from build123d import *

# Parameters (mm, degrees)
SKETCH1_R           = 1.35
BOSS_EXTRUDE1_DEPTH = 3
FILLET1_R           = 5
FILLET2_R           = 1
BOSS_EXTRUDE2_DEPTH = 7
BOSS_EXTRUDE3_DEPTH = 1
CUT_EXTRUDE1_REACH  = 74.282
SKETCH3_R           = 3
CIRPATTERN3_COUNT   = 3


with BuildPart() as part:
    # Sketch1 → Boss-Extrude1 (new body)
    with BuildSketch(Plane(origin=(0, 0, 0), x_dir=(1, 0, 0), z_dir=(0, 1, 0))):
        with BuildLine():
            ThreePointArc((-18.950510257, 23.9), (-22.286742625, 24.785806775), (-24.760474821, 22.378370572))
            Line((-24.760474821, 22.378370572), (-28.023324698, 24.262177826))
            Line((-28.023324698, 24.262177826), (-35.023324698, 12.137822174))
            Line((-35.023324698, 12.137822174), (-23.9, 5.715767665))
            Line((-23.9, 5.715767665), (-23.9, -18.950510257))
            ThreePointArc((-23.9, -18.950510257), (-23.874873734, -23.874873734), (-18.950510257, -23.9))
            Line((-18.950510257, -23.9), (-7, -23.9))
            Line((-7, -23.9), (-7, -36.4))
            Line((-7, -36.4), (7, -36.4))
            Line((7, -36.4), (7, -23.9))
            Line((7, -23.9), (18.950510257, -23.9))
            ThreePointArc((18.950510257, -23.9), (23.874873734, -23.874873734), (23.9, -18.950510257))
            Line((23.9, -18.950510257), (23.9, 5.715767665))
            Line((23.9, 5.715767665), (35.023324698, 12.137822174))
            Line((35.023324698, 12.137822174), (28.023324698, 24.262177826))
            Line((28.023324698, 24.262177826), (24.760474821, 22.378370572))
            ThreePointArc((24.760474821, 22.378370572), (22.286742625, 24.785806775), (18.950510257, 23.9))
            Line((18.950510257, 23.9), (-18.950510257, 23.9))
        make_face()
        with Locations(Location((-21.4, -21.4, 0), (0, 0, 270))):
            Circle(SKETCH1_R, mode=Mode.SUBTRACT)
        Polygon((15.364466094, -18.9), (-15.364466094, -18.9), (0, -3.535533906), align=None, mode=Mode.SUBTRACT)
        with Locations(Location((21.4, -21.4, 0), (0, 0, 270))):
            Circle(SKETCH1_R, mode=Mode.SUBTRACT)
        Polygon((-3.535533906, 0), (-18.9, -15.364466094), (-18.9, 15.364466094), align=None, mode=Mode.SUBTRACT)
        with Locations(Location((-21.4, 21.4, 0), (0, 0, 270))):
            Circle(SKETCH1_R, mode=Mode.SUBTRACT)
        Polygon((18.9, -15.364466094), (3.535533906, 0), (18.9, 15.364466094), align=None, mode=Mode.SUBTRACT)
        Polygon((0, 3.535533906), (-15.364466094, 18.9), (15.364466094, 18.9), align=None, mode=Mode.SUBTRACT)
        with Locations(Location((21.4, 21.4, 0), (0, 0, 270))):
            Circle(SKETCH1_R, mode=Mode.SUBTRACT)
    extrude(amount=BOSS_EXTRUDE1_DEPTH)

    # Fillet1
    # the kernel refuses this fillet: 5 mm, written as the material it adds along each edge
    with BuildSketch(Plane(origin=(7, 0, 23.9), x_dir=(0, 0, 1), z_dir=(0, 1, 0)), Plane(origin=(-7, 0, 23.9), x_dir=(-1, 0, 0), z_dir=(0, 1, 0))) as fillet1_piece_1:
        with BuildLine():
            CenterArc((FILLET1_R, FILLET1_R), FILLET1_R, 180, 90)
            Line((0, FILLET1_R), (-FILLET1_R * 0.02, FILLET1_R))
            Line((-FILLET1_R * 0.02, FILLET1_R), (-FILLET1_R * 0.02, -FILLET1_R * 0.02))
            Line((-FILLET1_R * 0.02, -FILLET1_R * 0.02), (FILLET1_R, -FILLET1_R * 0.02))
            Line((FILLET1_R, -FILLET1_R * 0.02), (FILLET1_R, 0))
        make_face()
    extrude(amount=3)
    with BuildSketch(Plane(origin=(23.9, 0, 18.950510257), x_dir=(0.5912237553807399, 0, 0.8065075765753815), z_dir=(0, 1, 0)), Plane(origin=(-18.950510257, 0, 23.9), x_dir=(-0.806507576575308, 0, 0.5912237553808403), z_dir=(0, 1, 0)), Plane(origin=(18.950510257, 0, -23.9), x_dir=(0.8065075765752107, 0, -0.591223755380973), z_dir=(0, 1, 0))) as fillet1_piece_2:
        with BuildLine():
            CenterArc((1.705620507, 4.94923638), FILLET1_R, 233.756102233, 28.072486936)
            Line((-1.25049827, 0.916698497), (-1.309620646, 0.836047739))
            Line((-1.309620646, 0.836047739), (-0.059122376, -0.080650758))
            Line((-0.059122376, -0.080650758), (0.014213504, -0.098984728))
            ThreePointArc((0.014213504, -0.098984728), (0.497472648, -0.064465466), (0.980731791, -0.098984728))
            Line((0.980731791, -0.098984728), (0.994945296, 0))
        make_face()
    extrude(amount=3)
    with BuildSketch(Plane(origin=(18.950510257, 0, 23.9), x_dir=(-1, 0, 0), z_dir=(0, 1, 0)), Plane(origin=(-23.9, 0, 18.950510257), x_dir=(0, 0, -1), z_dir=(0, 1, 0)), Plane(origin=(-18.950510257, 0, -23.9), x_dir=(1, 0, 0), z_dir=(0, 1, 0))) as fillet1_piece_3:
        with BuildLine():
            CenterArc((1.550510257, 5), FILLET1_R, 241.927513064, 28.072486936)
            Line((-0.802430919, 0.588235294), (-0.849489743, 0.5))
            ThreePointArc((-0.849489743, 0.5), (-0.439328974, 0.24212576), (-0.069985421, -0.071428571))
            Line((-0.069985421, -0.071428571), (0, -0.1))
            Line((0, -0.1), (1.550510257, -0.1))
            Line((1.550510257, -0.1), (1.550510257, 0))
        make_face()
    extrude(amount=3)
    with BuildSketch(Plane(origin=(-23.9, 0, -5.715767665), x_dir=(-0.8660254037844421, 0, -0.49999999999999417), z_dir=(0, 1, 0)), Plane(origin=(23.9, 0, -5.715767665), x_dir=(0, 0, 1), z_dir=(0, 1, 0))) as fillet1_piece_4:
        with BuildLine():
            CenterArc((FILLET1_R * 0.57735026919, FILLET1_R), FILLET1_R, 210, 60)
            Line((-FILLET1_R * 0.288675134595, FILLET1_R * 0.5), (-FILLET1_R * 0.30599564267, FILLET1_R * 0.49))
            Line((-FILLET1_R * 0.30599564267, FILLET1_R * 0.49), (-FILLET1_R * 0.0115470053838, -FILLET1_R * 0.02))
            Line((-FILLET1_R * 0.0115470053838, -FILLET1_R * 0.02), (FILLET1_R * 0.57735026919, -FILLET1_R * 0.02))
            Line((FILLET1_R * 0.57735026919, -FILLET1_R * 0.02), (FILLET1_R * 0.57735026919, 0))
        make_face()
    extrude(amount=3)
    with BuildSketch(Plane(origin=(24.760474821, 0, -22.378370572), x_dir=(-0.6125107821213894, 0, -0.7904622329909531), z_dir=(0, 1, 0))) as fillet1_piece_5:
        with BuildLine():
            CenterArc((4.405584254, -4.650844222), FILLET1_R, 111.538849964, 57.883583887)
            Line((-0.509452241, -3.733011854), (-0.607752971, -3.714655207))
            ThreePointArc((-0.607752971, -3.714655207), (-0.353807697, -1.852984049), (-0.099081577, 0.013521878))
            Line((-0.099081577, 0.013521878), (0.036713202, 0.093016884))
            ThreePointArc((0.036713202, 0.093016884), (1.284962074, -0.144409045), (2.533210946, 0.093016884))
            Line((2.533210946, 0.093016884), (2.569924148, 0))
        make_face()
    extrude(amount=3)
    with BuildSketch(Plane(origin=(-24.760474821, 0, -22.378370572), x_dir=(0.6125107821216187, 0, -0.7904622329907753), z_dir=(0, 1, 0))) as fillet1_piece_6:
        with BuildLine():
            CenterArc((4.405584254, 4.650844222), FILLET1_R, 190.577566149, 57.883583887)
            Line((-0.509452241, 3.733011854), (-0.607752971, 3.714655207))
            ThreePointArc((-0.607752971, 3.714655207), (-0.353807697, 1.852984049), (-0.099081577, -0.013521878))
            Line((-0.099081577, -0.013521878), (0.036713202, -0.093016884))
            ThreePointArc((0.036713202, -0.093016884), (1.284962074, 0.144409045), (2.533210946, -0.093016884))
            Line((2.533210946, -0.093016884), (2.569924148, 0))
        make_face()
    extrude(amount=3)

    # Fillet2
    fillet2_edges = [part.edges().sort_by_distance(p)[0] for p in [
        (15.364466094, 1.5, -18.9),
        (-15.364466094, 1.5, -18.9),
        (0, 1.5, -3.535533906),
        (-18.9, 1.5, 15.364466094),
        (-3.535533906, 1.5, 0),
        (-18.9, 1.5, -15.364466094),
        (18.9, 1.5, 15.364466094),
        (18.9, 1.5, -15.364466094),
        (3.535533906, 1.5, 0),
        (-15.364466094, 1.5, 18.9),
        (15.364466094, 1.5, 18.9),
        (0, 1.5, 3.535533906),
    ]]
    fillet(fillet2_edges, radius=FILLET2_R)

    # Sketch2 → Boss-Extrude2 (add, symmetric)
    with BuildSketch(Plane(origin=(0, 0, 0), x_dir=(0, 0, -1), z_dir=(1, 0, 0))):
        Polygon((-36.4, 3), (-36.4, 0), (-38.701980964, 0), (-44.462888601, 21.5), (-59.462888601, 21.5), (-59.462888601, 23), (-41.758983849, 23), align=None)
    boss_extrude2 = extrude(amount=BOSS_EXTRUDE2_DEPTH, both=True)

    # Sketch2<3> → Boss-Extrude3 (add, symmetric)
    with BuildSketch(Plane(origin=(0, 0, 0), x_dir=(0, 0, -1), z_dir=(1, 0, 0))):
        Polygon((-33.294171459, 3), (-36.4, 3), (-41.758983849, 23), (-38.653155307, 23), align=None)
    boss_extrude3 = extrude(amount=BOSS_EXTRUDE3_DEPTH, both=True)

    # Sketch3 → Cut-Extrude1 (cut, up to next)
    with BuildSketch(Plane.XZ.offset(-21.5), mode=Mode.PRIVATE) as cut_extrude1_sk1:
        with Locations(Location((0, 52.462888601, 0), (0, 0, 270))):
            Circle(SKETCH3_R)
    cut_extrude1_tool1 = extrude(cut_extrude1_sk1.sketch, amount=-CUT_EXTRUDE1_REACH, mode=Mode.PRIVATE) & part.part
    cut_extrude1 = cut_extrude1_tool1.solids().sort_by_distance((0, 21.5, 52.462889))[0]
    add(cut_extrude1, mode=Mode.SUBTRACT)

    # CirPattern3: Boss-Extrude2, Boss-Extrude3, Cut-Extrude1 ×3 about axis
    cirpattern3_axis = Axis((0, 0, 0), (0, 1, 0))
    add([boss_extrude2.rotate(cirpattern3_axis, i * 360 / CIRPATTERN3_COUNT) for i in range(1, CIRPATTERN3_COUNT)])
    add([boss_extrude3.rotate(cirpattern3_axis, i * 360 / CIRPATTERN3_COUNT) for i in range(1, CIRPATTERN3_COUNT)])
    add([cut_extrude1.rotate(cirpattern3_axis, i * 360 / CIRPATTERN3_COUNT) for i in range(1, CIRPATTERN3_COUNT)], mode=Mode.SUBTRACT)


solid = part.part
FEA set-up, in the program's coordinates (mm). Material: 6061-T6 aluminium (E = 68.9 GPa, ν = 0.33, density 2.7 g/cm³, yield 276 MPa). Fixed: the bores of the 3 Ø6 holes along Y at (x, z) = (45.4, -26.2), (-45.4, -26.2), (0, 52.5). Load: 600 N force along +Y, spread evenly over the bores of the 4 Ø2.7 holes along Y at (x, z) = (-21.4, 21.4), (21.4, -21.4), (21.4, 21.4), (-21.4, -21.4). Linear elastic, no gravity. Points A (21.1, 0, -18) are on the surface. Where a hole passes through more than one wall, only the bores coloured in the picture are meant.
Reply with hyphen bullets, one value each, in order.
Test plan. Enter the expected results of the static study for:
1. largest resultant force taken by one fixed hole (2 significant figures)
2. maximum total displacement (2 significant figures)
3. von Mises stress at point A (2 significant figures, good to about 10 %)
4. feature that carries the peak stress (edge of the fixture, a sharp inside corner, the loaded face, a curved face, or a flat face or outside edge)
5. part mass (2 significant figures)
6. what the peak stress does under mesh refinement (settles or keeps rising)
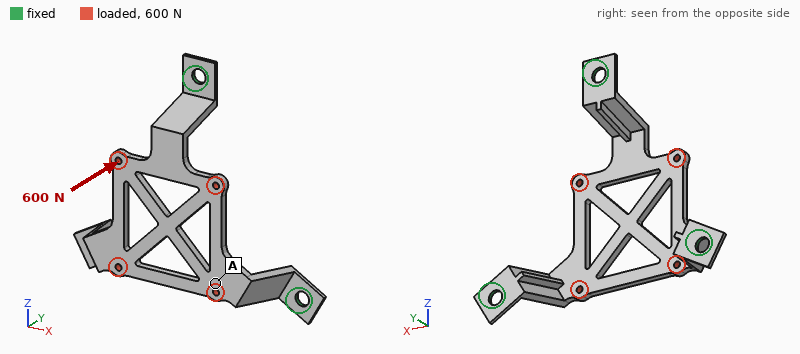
- 280 N
- 0.32 mm
- 27 MPa
- edge of the fixture
- 26 g
- keeps rising
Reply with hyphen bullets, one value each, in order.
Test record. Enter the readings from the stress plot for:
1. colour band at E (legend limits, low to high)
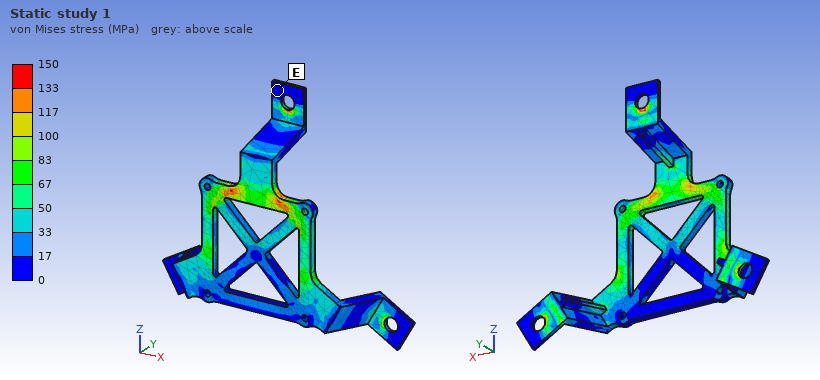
- 0 to 17 MPa
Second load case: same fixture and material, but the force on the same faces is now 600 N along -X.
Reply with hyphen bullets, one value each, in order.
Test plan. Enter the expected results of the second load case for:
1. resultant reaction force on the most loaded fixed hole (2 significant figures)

- 260 N
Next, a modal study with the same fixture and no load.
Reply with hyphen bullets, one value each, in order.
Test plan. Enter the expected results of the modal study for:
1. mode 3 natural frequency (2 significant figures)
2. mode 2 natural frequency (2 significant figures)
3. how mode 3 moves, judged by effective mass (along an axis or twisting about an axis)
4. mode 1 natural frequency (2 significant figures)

- 2400 Hz
- 1700 Hz
- twisting about Y
- 1600 Hz
